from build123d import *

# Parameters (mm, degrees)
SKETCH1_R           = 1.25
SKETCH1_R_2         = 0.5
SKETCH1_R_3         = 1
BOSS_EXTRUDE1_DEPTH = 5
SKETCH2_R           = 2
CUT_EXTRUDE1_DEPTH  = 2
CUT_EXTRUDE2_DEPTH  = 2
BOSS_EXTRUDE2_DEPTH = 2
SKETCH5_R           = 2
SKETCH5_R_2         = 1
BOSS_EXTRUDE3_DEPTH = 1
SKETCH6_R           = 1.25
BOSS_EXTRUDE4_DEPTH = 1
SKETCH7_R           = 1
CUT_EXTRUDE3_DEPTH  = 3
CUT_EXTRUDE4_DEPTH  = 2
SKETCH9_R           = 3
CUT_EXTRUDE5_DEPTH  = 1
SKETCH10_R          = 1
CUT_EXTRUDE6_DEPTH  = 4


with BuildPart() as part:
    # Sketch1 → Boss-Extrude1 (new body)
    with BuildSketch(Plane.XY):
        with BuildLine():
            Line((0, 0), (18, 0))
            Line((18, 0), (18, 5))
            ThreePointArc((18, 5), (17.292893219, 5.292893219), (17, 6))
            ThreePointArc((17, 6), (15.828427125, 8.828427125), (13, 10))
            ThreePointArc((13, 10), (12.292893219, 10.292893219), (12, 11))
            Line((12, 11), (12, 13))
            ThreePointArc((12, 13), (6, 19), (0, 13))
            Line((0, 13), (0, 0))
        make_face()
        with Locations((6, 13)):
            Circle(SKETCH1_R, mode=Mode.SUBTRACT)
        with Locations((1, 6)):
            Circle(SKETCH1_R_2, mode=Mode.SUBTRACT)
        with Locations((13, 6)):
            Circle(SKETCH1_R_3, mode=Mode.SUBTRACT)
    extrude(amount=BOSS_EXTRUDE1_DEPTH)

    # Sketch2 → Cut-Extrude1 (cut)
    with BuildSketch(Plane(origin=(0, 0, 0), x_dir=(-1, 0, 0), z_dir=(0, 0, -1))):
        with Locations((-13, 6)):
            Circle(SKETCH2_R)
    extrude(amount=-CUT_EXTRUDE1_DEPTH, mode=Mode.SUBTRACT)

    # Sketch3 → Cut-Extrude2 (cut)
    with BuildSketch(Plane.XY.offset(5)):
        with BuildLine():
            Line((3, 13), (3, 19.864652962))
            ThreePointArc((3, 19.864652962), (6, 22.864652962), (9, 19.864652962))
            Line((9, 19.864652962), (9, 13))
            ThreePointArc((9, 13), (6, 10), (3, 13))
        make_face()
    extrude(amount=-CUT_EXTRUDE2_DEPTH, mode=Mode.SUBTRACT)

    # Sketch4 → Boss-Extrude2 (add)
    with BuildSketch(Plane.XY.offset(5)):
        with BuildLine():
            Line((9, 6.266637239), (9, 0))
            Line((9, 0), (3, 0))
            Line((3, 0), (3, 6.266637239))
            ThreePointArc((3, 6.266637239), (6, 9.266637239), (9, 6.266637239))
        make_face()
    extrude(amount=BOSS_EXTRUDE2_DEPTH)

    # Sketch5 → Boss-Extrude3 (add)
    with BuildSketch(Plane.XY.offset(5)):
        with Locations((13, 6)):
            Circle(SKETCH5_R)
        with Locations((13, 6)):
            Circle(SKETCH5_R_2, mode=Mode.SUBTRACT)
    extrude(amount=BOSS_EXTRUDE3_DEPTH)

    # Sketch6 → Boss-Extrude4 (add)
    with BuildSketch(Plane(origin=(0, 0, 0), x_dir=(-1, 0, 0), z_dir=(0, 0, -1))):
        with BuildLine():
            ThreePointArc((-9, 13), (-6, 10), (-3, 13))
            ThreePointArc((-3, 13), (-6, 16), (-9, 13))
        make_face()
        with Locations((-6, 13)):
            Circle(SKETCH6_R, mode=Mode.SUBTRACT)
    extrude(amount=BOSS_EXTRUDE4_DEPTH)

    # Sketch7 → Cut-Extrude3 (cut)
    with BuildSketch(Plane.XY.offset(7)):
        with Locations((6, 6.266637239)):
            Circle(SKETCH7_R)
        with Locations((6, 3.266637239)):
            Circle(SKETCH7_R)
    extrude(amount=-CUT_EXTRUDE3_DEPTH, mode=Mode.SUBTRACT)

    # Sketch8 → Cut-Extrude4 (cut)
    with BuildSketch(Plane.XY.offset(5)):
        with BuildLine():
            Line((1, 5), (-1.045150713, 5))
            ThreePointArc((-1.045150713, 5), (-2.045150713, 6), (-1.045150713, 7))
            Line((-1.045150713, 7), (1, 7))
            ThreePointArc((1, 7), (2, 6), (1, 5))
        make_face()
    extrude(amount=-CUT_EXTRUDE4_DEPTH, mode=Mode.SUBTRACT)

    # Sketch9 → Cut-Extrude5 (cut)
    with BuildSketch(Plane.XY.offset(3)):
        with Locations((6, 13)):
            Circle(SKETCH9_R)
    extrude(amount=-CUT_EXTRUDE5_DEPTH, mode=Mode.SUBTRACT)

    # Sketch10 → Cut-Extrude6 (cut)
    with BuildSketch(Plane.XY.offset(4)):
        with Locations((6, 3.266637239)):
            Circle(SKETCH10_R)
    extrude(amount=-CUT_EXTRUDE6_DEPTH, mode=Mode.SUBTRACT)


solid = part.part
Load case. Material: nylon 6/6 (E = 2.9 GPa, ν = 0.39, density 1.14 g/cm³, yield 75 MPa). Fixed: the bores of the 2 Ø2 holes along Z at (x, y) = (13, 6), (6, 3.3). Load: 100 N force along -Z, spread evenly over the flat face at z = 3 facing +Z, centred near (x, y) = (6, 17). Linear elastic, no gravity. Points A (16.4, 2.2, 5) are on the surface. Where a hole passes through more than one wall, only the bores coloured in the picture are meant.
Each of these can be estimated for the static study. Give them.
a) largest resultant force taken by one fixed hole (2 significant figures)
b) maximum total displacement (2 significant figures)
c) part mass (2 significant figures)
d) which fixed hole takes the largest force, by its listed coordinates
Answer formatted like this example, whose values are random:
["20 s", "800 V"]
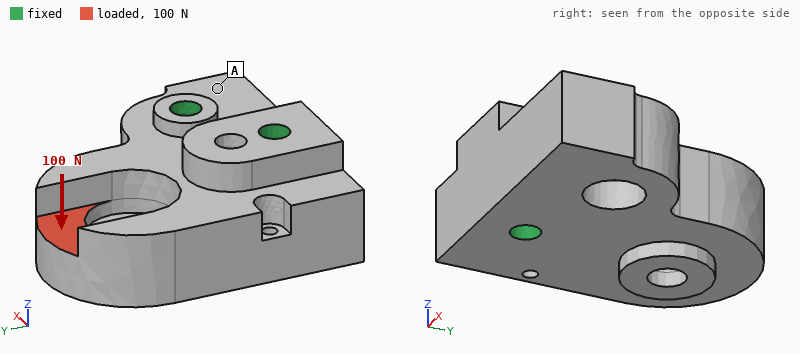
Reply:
["62 N", "0.33 mm", "1.4 g", "(6, 3.3)"]
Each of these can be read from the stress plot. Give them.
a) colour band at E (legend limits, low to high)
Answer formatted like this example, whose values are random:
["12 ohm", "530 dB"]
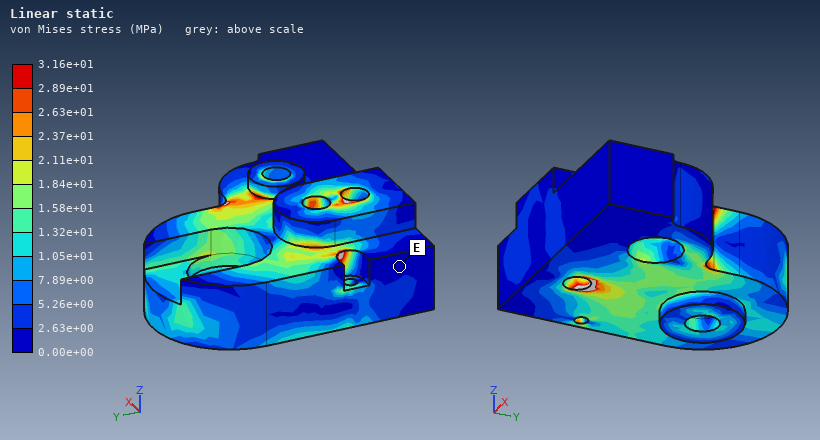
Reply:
["0.00e+00 to 2.63e+00 MPa"]
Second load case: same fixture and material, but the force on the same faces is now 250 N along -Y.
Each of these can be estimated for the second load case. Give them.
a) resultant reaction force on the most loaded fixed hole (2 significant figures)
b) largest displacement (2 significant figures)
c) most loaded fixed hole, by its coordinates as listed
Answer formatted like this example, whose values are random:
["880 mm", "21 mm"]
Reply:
["220 N", "0.18 mm", "(6, 3.3)"]
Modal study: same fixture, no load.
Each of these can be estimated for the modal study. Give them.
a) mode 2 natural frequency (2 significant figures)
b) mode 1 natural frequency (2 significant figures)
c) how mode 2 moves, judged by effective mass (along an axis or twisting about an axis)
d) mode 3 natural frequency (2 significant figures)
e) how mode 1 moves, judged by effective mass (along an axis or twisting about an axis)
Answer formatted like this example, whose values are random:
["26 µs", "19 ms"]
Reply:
["11 kHz", "7000 Hz", "along X", "14 kHz", "along Z"]
